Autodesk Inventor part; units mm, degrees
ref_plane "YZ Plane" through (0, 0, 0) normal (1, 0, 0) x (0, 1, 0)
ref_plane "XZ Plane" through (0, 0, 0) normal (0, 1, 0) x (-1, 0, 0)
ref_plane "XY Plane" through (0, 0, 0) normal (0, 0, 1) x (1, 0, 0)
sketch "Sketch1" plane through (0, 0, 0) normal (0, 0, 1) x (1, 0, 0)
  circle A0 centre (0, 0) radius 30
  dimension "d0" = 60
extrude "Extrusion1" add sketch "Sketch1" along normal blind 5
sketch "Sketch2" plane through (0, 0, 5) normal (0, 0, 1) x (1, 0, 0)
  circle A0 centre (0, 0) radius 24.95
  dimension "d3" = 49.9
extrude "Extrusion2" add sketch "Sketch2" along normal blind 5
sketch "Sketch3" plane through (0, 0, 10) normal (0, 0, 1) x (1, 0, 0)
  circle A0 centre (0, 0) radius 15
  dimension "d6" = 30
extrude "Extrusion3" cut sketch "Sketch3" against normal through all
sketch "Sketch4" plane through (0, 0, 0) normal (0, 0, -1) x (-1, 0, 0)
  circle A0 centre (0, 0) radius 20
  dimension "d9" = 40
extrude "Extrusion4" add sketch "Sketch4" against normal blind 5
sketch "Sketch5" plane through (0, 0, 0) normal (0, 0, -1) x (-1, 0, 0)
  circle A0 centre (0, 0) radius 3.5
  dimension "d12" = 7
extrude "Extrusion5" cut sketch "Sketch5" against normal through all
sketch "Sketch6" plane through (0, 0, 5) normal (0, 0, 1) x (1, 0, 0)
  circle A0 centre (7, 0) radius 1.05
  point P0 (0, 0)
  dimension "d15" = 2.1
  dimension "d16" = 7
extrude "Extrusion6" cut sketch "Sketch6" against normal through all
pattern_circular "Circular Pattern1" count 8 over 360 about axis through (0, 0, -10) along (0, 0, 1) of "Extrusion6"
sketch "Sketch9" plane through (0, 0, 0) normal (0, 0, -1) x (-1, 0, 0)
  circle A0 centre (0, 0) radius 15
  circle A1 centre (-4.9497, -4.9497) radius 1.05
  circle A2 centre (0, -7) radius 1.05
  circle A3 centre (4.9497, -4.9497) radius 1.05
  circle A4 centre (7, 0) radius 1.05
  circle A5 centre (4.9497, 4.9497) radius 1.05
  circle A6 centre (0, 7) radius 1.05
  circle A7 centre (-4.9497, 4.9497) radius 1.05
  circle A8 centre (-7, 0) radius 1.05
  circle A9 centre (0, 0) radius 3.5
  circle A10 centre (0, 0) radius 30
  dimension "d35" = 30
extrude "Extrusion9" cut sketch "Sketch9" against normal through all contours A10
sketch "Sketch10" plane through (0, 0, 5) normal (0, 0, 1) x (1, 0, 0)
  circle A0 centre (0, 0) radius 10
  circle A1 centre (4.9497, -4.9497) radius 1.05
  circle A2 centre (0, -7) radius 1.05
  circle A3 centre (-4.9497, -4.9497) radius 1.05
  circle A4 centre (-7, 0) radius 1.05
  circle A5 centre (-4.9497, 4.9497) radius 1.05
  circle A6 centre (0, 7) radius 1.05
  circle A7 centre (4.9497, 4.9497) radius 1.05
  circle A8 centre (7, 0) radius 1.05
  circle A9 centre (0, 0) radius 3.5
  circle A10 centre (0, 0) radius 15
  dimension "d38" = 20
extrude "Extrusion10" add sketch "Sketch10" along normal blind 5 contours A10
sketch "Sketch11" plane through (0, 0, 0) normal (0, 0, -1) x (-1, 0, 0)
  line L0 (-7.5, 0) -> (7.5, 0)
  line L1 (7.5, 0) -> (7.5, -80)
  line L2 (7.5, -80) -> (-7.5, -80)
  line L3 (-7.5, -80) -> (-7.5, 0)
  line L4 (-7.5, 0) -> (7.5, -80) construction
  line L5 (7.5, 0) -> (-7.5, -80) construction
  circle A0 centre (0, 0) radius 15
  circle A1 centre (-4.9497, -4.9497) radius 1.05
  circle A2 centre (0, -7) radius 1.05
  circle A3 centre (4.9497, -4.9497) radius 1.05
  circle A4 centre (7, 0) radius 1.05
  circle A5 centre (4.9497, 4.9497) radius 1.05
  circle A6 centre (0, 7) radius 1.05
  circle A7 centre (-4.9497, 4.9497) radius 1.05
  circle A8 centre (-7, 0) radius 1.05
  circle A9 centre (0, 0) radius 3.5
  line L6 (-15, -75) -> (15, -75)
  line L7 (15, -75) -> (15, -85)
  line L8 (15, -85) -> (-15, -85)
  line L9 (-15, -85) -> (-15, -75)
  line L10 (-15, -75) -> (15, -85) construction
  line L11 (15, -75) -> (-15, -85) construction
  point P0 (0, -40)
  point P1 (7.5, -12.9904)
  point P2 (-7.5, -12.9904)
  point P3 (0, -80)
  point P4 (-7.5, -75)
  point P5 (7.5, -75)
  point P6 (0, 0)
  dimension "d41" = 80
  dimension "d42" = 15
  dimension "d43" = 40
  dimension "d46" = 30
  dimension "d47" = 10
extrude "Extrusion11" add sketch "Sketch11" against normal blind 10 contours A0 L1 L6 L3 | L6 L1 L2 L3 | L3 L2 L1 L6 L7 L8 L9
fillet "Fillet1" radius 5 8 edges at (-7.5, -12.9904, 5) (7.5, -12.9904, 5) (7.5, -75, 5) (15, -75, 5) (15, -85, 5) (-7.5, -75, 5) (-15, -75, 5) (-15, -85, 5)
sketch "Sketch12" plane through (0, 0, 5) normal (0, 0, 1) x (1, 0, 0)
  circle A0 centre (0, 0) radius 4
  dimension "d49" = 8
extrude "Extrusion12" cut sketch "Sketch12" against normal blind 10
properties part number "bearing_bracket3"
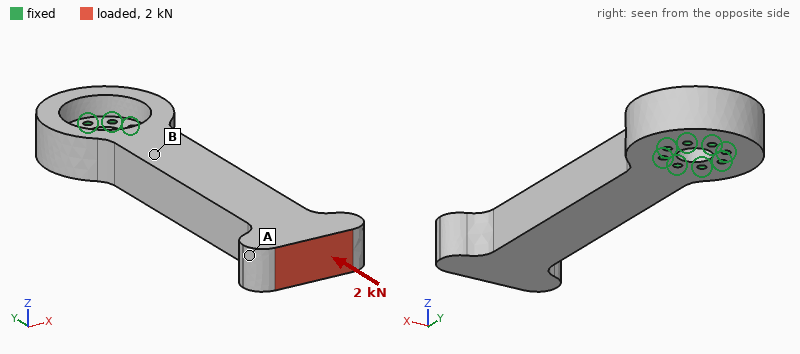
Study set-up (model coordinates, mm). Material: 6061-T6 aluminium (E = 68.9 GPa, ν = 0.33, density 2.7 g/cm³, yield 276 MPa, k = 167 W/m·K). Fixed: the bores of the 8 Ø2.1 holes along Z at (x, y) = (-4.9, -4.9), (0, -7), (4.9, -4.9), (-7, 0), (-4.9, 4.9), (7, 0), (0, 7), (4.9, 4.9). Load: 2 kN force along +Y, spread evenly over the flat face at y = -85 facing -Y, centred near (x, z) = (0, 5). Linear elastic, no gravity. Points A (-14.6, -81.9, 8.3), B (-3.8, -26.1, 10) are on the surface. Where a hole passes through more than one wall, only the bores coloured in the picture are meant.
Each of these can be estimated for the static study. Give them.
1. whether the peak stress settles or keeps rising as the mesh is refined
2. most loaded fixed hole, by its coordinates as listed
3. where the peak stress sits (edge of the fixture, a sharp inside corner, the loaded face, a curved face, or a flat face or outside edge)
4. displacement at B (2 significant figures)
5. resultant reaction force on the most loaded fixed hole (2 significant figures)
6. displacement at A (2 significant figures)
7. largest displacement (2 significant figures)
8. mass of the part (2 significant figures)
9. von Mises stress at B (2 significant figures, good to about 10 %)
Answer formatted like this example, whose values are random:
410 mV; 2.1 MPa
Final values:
keeps rising; (0, -7); edge of the fixture; 17 µm; 590 N; 58 µm; 61 µm; 46 g; 13 MPa
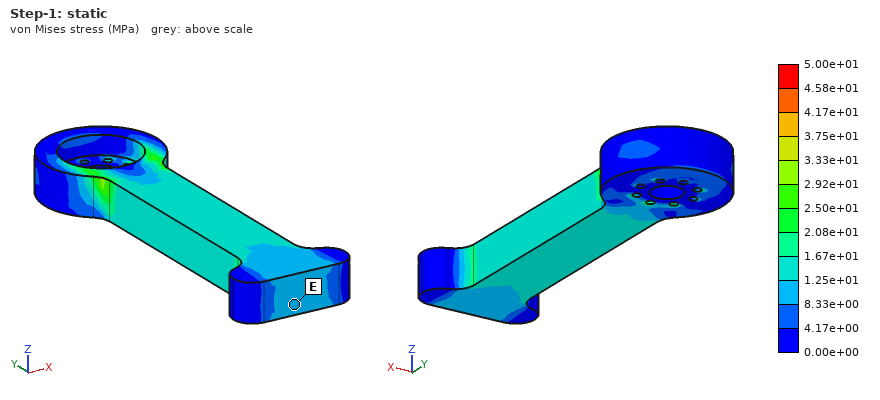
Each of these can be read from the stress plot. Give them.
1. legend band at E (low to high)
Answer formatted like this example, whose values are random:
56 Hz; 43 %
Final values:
8.33e+00 to 1.25e+01 MPa
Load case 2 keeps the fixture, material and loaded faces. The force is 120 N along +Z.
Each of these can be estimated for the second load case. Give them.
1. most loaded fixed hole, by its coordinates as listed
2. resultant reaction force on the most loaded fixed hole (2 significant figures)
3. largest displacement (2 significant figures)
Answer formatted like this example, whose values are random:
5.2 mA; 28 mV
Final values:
(0, -7); 430 N; 0.31 mm
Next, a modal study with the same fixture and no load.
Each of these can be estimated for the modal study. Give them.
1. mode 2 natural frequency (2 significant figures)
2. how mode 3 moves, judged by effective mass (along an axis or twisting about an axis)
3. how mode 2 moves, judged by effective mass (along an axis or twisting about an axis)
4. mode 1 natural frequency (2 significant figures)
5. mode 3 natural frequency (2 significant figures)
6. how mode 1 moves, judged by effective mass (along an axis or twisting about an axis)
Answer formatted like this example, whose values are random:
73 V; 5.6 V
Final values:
1600 Hz; twisting about Y; along X; 930 Hz; 5600 Hz; along Z
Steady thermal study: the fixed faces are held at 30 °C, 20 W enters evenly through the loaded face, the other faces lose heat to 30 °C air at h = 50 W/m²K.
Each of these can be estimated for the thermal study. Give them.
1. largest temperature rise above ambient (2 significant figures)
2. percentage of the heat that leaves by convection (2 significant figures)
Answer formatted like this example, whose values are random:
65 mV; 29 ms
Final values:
48 K; 29 %
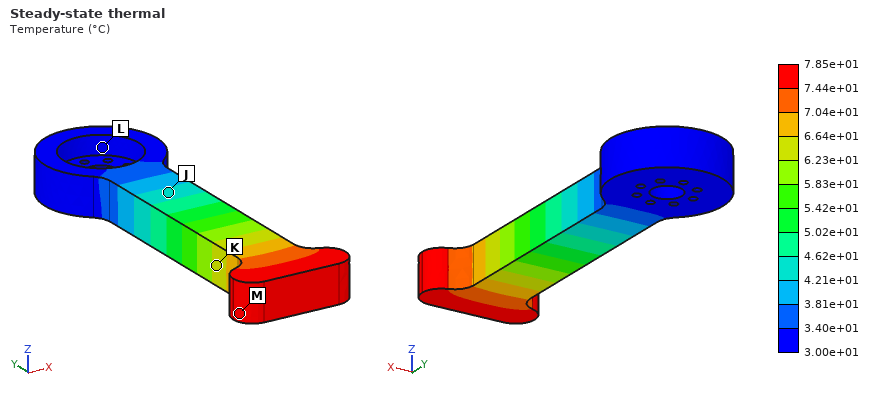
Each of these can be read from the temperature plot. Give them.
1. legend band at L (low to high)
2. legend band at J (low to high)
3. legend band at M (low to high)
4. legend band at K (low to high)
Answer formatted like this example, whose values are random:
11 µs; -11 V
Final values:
3.00e+01 to 3.40e+01 °C; 4.21e+01 to 4.62e+01 °C; 7.44e+01 to 7.85e+01 °C; 6.23e+01 to 6.64e+01 °C
